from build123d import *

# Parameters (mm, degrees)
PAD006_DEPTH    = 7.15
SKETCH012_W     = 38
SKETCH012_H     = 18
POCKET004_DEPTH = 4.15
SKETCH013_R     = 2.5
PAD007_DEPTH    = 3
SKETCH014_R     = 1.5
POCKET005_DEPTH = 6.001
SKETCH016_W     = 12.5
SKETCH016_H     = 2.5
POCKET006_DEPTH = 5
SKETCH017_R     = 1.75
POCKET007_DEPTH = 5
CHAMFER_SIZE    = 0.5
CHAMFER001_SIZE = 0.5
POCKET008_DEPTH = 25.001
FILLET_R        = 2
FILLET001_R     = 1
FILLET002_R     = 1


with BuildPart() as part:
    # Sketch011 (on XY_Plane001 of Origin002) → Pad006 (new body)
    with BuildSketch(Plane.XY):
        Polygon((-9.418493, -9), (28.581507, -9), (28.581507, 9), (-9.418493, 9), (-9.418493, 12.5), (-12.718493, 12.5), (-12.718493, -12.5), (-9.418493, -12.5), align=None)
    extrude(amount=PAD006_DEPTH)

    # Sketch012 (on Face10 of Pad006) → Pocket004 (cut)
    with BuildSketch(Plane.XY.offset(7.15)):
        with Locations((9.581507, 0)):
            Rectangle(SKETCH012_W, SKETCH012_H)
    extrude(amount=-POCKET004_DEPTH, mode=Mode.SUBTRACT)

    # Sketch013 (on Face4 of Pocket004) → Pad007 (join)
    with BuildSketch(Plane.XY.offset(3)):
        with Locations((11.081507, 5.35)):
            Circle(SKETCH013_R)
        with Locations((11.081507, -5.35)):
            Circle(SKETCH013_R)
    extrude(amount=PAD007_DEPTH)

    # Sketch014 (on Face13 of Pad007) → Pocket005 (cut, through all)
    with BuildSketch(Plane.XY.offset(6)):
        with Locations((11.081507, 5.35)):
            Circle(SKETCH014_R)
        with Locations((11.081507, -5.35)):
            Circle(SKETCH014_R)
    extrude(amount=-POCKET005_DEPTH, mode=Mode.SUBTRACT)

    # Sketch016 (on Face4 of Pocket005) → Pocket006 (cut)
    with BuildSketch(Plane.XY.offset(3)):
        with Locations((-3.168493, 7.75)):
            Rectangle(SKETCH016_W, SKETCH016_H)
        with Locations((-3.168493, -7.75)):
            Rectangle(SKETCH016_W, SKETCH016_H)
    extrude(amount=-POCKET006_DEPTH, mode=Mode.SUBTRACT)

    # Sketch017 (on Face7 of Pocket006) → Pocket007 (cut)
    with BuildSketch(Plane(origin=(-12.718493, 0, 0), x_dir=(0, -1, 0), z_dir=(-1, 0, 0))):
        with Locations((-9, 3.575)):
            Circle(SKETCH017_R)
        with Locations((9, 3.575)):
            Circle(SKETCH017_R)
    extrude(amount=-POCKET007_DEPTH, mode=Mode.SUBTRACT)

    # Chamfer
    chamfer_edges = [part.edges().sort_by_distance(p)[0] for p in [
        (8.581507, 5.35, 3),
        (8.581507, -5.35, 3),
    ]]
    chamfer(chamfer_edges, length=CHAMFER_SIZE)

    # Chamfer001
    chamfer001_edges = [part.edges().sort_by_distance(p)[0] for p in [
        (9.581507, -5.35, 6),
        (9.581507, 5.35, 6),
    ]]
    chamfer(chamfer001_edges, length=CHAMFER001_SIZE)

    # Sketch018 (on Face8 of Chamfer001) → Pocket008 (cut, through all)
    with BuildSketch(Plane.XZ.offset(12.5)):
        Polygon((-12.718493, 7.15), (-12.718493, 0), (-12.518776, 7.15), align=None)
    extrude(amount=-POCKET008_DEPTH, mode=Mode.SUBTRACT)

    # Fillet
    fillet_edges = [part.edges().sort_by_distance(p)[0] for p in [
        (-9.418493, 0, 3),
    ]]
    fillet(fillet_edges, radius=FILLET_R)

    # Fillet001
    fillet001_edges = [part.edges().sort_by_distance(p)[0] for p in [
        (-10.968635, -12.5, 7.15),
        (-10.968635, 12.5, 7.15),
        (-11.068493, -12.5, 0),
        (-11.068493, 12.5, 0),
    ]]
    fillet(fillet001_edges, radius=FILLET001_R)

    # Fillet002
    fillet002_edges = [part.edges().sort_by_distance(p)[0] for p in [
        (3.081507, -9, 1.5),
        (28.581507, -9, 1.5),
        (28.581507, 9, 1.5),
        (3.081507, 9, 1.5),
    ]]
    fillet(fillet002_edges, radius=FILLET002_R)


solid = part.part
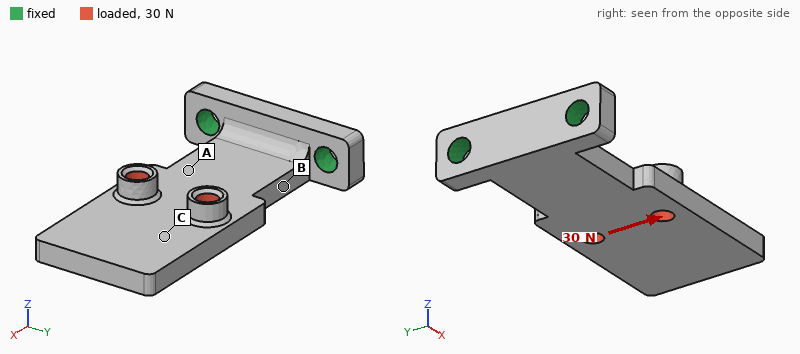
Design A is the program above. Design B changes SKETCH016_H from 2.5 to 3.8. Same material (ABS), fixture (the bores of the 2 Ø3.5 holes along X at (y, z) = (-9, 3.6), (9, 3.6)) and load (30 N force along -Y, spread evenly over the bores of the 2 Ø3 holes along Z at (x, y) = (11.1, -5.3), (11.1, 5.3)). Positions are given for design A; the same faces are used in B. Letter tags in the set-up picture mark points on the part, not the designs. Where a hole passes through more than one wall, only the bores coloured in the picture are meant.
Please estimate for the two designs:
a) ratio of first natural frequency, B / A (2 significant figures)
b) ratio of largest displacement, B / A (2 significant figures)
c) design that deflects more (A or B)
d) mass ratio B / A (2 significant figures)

0.95
1.3
B
0.98
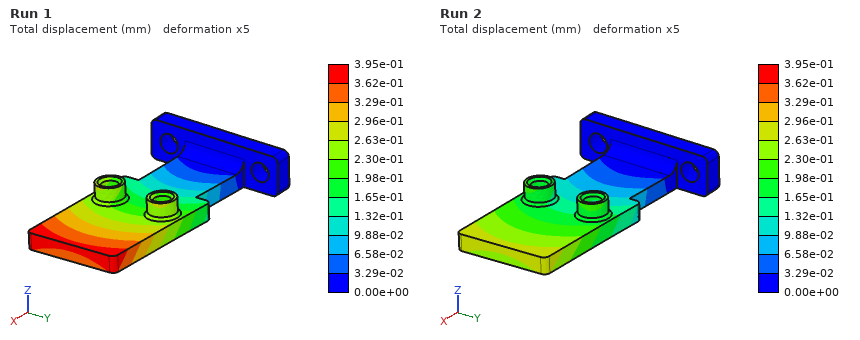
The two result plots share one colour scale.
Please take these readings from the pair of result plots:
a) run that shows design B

Run 1
